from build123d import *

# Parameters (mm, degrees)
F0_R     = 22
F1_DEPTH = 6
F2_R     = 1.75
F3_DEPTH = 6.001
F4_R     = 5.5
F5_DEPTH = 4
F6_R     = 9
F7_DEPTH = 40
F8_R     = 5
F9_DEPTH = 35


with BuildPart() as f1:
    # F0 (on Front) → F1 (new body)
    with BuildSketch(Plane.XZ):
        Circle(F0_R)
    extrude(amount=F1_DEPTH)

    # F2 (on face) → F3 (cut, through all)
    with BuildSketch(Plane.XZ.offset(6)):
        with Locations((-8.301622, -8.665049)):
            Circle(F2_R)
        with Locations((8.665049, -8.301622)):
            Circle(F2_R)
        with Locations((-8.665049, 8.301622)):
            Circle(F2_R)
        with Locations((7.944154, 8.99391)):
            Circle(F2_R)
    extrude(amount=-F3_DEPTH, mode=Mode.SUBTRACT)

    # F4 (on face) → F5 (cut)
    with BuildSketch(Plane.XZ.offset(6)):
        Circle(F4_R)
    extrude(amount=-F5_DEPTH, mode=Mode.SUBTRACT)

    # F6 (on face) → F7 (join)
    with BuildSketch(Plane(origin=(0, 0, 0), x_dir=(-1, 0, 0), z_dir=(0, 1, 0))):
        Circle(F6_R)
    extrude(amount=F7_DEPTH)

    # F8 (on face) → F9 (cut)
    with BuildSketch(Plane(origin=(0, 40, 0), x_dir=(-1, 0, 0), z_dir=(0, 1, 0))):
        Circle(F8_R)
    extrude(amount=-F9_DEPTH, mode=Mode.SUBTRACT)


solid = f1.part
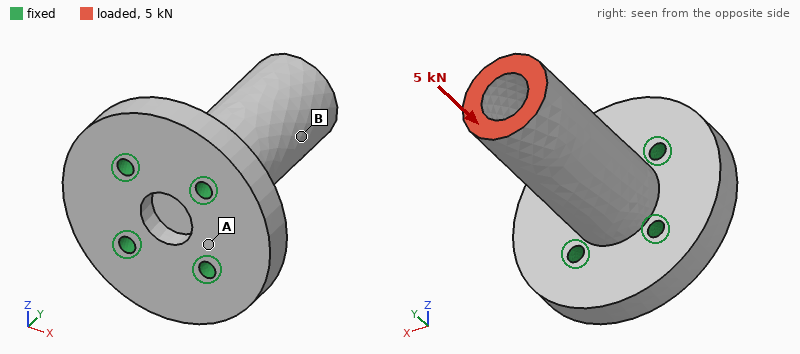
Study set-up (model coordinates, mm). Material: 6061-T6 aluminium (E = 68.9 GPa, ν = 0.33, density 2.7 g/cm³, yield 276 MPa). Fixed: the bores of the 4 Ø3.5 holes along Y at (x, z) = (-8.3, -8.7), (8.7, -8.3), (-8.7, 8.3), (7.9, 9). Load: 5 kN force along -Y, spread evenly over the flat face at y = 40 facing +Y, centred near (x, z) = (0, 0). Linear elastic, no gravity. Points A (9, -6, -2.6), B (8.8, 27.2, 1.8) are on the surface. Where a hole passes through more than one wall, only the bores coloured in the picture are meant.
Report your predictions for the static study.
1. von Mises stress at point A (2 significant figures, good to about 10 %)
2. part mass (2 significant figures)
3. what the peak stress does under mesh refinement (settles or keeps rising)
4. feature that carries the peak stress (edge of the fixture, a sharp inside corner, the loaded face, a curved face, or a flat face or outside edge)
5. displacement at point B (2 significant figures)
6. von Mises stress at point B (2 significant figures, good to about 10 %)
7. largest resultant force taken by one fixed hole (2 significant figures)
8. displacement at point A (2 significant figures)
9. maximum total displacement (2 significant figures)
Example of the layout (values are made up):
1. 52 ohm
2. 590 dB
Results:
1. 13 MPa
2. 43 g
3. keeps rising
4. edge of the fixture
5. 15 µm
6. 28 MPa
7. 1.4 kN
8. 3.2 µm
9. 21 µm
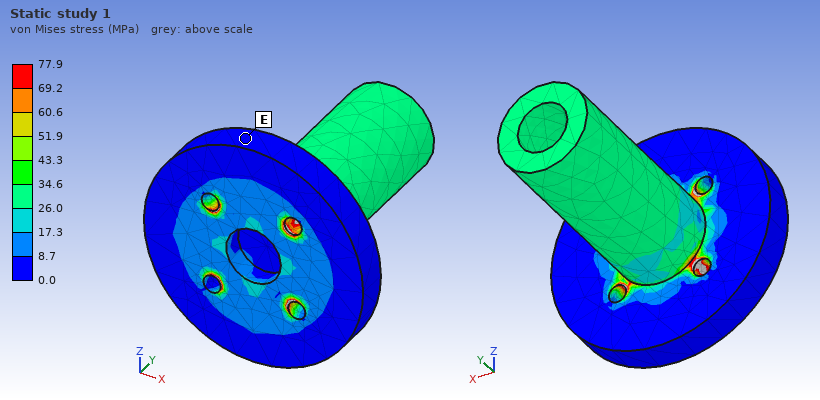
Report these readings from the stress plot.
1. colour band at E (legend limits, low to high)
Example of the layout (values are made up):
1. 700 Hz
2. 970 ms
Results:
1. 0.0 to 8.7 MPa
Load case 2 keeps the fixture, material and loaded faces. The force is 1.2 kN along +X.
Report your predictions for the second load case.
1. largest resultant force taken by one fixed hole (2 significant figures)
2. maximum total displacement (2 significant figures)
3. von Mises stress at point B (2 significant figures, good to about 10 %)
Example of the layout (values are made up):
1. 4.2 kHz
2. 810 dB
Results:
1. 1.7 kN
2. 0.14 mm
3. 30 MPa
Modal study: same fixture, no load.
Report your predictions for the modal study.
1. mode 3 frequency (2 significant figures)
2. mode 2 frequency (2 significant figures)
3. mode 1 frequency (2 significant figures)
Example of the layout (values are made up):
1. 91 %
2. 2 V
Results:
1. 18 kHz
2. 6400 Hz
3. 6400 Hz
